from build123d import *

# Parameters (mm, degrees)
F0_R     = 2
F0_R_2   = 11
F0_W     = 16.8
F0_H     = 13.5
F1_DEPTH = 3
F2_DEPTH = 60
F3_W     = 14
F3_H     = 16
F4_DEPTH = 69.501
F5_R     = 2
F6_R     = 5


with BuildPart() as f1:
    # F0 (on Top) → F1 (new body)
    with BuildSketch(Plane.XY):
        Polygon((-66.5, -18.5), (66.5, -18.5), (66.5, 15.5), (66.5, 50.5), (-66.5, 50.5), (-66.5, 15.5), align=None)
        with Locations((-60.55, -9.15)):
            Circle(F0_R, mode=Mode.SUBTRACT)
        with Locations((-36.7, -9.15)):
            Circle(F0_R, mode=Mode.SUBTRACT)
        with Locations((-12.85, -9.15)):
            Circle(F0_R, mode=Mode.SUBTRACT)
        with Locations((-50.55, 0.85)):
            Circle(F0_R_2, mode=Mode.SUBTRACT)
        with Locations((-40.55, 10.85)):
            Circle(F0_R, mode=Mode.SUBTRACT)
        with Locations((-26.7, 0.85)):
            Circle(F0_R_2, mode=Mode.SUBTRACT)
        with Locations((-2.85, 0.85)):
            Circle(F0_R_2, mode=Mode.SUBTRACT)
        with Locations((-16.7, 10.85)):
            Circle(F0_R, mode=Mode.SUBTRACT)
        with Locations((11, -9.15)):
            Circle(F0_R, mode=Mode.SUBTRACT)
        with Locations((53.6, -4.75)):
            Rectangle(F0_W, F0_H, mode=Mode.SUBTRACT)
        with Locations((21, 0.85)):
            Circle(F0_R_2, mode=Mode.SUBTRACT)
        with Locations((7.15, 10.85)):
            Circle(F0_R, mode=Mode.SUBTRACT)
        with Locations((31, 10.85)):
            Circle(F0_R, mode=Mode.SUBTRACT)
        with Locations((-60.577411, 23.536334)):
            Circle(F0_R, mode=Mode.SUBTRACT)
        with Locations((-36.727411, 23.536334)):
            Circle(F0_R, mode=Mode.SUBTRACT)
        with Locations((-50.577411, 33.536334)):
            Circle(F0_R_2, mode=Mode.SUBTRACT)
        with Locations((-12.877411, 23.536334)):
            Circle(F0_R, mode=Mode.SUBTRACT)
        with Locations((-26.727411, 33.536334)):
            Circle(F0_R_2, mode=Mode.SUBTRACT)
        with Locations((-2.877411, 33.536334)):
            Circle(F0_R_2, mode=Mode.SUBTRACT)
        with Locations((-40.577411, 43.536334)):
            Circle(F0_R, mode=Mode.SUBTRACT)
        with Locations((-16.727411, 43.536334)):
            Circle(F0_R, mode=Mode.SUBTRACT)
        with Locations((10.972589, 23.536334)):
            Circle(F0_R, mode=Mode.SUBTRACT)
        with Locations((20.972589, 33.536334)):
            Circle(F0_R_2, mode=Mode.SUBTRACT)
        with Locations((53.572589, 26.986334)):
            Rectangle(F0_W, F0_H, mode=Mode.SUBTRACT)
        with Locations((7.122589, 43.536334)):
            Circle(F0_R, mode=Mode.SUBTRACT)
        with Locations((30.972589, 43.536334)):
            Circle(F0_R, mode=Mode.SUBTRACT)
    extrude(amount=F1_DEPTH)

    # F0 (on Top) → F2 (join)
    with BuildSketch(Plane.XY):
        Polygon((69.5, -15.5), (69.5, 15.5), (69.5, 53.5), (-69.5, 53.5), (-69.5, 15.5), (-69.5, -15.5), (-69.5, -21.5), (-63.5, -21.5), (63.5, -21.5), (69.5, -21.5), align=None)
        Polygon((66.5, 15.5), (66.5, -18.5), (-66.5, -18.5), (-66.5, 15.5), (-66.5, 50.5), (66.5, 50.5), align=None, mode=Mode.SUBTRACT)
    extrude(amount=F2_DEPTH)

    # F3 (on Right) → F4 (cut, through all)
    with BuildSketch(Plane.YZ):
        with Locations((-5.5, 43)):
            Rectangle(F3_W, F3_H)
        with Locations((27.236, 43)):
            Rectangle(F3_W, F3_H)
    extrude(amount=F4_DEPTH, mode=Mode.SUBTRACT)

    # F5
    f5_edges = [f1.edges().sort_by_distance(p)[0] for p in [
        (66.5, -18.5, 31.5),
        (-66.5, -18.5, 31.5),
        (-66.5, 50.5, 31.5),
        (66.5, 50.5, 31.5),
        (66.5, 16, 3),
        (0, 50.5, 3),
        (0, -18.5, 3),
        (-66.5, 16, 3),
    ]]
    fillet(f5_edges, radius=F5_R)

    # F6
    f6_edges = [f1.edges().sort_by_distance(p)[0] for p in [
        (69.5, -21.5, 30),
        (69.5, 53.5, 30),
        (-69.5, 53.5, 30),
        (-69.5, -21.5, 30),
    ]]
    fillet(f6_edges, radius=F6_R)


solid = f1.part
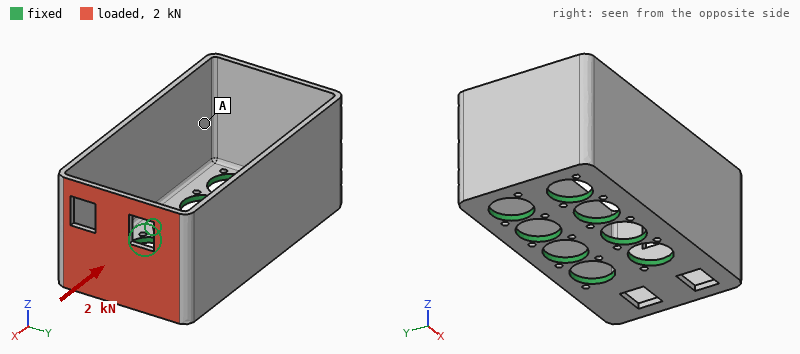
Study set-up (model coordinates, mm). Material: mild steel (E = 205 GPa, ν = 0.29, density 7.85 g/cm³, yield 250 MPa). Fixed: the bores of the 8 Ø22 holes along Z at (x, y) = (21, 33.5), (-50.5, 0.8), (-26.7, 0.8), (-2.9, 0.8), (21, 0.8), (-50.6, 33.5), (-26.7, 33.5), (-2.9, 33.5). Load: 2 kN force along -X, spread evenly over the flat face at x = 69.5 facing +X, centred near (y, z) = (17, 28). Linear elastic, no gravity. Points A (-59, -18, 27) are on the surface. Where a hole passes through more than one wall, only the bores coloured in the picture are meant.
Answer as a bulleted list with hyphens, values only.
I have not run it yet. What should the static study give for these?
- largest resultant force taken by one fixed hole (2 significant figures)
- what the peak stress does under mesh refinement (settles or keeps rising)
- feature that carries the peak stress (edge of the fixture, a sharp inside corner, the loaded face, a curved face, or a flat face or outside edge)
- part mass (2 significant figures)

- 620 N
- keeps rising
- a sharp inside corner
- 700 g
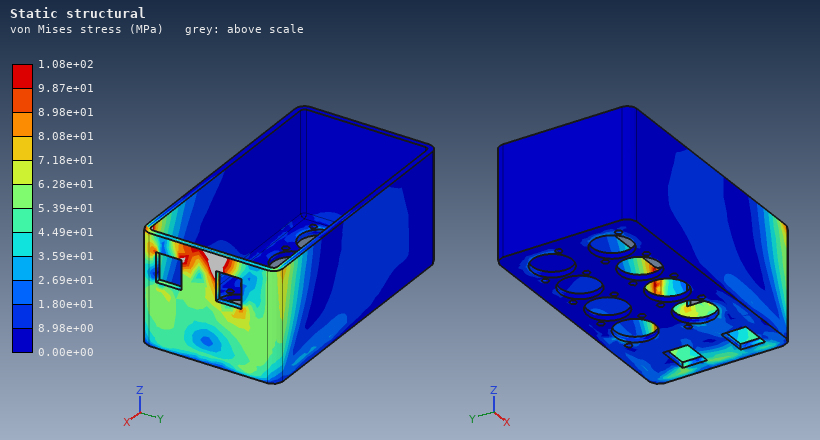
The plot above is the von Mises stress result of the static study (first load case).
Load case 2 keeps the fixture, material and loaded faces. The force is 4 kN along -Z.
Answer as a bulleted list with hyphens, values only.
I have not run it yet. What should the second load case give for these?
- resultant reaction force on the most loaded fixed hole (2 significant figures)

- 2.9 kN
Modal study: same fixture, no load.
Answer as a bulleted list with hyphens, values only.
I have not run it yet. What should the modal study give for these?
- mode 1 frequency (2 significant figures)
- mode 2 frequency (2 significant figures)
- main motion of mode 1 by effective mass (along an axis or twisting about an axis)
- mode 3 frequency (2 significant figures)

- 1000 Hz
- 1100 Hz
- along Y
- 1700 Hz
